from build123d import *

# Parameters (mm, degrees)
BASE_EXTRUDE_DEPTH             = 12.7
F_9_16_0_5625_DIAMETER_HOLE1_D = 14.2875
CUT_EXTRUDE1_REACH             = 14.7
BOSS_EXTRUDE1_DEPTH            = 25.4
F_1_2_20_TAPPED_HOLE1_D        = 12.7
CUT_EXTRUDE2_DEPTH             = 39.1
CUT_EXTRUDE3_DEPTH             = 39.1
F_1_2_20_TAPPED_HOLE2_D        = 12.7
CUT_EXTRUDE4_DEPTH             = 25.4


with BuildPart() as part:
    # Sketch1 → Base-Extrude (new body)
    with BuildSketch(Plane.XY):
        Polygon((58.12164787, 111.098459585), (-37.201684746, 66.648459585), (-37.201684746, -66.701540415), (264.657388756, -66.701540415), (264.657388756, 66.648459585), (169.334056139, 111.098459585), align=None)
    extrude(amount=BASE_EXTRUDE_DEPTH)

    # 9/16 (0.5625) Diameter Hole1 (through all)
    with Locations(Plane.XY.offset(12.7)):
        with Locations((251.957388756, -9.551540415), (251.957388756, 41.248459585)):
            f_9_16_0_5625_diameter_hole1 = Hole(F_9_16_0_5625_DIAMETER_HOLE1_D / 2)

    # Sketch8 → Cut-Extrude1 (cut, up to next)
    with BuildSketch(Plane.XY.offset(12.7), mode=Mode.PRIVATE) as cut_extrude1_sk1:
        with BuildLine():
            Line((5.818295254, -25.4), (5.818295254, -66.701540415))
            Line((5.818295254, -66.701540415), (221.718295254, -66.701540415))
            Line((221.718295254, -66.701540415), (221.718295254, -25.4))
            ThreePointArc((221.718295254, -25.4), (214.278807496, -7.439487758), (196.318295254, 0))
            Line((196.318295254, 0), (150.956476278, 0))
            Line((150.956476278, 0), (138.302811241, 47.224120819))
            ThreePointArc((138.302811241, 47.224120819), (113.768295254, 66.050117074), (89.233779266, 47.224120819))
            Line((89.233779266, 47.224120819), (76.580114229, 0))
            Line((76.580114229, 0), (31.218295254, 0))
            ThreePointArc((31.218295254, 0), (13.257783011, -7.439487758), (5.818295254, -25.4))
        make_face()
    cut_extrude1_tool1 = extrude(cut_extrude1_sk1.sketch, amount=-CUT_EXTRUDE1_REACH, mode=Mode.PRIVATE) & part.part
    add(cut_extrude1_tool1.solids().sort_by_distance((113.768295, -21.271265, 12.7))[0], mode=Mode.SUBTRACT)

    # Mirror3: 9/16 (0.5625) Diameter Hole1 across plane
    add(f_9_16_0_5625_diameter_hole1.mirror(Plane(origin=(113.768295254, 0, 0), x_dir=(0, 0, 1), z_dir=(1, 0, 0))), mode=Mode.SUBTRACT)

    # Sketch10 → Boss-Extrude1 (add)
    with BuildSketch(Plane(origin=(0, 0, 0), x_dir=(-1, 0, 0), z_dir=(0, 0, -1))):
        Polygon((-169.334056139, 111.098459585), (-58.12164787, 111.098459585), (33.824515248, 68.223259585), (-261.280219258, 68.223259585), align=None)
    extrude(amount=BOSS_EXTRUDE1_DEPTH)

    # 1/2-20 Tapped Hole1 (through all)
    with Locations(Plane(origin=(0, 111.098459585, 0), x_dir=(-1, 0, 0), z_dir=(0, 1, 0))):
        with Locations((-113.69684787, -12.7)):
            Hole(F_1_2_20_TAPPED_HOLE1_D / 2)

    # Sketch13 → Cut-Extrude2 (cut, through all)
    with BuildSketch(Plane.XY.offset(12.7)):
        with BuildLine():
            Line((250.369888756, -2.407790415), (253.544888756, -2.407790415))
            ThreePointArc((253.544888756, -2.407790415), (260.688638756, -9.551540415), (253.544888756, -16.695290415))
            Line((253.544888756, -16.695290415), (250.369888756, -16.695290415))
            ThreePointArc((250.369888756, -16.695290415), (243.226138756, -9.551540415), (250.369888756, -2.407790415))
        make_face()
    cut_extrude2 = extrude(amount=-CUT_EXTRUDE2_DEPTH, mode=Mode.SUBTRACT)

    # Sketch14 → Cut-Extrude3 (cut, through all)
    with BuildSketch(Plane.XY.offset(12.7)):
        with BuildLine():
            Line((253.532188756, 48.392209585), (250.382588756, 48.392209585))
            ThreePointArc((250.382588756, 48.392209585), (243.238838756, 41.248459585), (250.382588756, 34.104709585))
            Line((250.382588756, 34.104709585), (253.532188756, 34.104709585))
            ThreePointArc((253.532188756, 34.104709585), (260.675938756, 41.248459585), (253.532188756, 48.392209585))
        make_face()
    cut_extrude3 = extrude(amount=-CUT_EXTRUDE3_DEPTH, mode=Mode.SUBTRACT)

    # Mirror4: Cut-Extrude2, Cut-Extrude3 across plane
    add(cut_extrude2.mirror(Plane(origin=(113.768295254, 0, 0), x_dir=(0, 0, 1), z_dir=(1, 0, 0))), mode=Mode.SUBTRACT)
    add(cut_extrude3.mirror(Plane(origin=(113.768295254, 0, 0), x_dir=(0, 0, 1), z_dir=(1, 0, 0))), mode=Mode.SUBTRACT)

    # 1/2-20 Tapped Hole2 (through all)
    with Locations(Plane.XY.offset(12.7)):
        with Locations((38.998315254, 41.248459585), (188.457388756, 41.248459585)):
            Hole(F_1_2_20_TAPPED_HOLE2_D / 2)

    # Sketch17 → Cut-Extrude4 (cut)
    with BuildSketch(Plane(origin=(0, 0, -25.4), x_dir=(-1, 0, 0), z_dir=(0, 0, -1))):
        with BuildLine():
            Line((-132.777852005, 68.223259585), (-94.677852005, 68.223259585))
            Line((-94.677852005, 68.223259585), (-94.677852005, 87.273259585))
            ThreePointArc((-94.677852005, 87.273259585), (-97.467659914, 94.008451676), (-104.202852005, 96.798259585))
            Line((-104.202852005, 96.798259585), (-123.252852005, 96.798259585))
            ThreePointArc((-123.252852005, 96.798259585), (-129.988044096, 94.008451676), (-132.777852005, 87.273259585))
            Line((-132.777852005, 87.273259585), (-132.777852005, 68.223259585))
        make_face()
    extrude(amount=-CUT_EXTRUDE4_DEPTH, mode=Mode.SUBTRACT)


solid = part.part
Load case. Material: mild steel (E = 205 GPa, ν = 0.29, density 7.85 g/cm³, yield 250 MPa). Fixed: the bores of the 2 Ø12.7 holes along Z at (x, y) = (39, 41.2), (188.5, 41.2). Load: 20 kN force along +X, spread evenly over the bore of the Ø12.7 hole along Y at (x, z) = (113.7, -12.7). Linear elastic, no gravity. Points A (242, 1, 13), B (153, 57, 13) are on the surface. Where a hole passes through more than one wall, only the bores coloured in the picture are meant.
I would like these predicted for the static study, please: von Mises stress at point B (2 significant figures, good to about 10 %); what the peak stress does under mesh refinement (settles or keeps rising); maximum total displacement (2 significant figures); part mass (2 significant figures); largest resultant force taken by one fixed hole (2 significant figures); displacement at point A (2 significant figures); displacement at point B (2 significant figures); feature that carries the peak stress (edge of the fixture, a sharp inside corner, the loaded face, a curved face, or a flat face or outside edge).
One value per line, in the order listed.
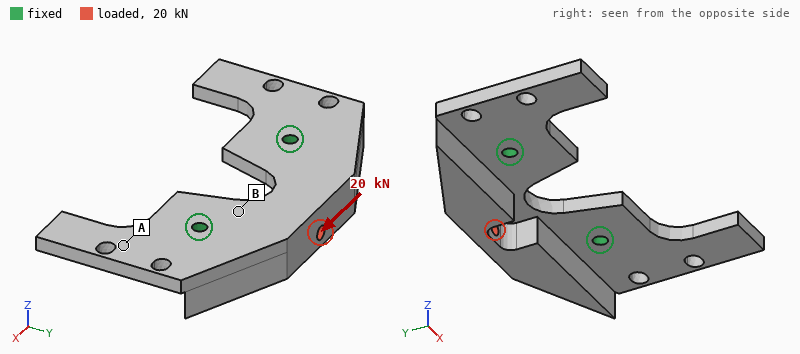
15 MPa
keeps rising
22 µm
4.6 kg
13 kN
9.2 µm
3.7 µm
edge of the fixture
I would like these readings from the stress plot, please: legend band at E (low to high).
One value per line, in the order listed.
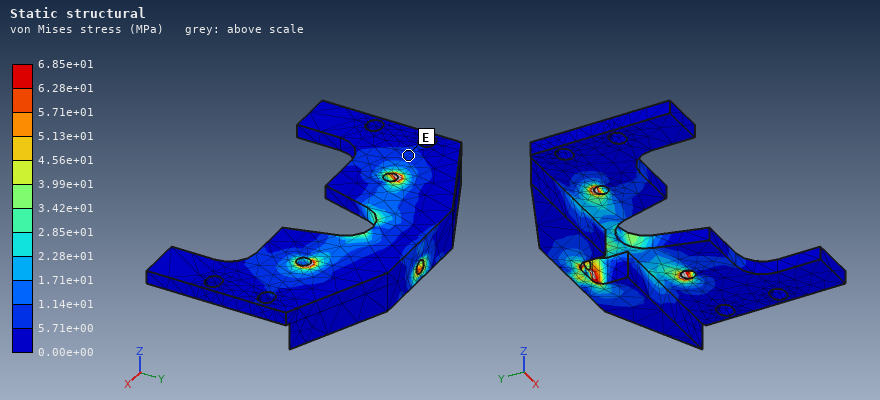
5.71e+00 to 1.14e+01 MPa
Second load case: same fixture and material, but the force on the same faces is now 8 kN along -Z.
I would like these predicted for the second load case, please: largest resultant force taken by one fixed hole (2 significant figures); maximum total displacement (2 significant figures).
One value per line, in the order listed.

4.0 kN
0.17 mm
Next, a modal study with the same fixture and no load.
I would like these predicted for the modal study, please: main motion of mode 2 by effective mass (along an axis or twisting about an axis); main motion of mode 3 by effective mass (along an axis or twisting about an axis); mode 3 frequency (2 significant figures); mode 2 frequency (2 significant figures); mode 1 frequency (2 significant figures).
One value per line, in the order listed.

twisting about Y
along Z
1200 Hz
830 Hz
790 Hz
